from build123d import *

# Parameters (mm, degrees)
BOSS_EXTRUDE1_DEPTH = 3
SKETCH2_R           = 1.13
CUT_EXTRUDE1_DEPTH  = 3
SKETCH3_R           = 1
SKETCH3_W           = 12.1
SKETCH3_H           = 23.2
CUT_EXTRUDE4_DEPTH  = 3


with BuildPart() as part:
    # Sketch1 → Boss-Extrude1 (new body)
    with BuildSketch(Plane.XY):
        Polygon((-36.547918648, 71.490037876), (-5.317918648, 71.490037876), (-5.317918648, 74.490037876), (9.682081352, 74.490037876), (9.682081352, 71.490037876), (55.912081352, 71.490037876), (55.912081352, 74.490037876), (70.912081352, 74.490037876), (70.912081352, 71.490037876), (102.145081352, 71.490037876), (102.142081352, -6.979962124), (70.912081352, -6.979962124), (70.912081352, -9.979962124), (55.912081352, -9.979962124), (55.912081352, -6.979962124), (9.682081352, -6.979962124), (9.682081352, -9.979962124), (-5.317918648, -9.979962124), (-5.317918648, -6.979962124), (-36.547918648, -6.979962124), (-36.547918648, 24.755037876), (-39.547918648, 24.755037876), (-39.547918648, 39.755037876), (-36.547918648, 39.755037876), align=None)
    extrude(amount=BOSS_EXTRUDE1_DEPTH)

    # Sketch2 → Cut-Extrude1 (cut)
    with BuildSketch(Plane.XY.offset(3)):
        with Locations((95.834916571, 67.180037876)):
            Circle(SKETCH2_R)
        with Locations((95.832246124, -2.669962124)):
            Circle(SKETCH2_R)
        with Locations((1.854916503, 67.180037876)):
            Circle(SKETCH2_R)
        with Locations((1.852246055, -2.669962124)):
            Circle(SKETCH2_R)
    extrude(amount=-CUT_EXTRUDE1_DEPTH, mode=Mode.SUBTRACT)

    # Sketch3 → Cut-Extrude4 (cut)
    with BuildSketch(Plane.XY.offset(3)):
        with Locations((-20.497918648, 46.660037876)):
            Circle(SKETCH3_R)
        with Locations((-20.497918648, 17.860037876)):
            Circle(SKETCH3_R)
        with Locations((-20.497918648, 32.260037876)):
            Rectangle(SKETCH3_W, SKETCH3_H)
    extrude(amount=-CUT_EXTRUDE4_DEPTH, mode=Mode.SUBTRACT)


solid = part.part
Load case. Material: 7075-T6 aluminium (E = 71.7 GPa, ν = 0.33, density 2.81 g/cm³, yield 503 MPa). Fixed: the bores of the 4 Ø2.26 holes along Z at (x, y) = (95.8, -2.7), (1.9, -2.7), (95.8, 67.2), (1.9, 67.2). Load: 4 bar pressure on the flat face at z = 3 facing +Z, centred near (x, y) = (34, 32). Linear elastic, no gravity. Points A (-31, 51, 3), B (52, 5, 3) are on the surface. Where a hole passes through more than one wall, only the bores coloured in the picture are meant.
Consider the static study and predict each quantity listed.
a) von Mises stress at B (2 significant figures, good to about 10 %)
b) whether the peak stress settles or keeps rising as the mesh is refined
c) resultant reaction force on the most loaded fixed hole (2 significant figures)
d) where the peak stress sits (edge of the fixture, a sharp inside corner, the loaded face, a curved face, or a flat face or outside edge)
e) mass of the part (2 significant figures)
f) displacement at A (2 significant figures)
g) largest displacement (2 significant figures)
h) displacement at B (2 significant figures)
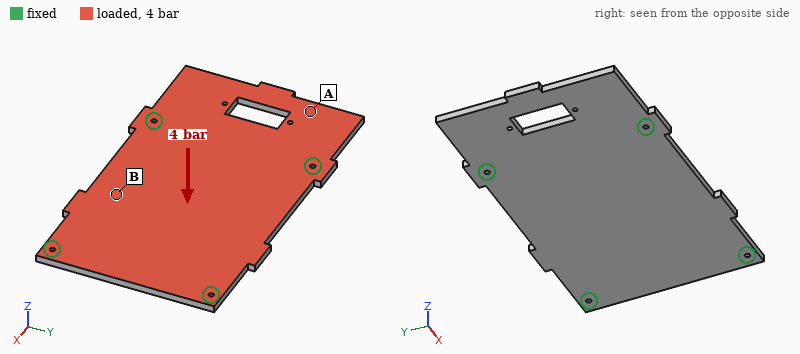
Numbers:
120 MPa
keeps rising
1.4 kN
edge of the fixture
91 g
0.73 mm
1.1 mm
0.77 mm
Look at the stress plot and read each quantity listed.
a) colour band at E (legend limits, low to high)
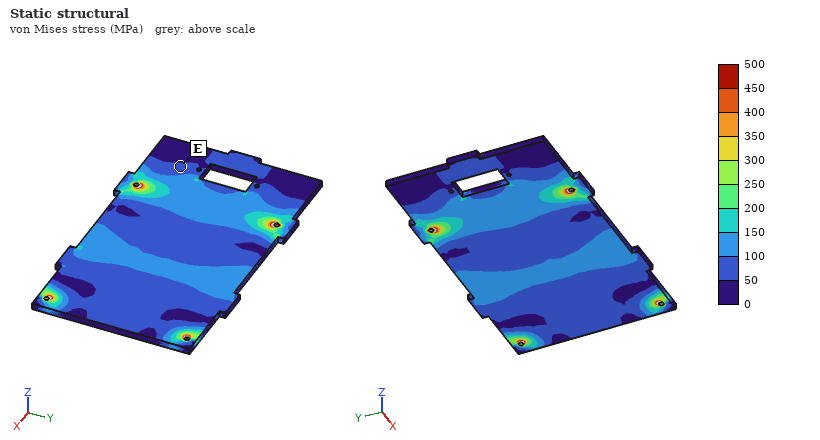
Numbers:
50 to 100 MPa
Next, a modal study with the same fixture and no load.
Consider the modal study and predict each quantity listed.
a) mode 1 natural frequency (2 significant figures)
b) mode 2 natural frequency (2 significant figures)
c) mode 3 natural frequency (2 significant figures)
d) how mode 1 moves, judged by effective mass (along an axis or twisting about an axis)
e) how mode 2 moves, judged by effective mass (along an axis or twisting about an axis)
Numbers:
1100 Hz
1400 Hz
2100 Hz
twisting about Y
along Z
